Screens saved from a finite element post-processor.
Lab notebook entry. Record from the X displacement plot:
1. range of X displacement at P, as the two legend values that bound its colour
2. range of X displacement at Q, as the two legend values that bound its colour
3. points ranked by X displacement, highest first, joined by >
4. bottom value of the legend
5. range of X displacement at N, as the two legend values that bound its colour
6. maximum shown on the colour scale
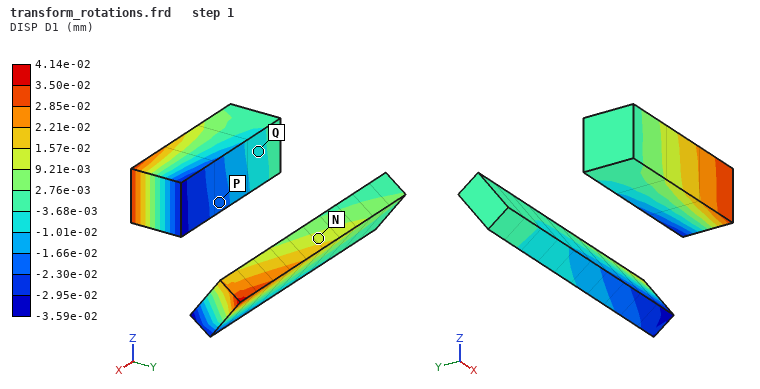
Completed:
-2.30e-02 to -1.66e-02 mm
-1.01e-02 to -3.68e-03 mm
N > Q > P
-3.59e-02 mm
9.21e-03 to 1.57e-02 mm
4.14e-02 mm
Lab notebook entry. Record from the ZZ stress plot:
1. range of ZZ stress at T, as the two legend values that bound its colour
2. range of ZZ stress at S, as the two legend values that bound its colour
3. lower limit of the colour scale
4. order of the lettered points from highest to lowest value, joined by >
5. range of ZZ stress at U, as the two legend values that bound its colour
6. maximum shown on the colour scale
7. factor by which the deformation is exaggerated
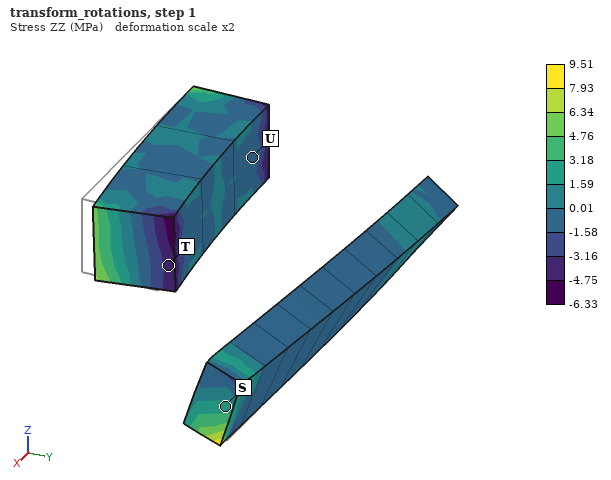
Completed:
-4.75 to -3.16 MPa
1.59 to 3.18 MPa
-6.33 MPa
S > U > T
-1.58 to 0.01 MPa
9.51 MPa
2
